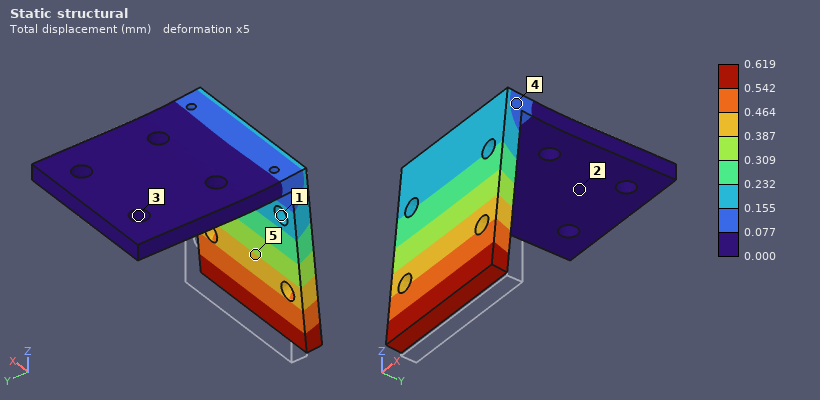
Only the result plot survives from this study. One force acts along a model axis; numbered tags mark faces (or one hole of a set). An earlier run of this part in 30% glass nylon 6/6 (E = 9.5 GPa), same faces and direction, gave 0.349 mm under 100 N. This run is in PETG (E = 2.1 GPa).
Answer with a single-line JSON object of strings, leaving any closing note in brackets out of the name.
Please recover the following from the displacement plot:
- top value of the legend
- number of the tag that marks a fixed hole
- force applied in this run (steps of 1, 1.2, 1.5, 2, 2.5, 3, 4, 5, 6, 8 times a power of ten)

{"top value of the legend": "0.619 mm", "number of the tag that marks a fixed hole": "3", "force applied in this run": "40 N"}
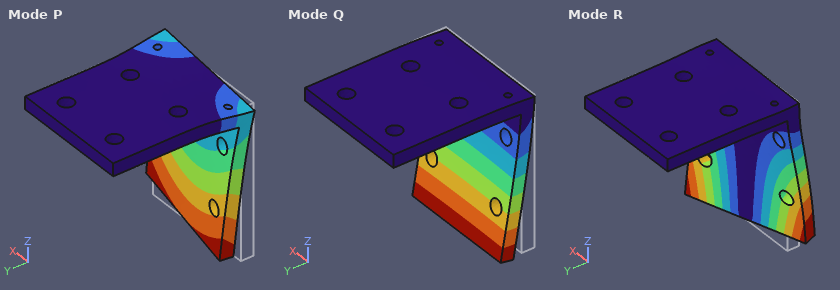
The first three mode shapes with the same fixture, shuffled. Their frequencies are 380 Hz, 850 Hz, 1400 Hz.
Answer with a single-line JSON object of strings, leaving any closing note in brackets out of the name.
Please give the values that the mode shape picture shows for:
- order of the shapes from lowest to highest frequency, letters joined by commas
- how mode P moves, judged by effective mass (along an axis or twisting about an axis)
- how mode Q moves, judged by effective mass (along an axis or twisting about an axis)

{"order of the shapes from lowest to highest frequency, letters joined by commas": "Q, P, R", "how mode P moves, judged by effective mass": "along X", "how mode Q moves, judged by effective mass": "along Y"}
